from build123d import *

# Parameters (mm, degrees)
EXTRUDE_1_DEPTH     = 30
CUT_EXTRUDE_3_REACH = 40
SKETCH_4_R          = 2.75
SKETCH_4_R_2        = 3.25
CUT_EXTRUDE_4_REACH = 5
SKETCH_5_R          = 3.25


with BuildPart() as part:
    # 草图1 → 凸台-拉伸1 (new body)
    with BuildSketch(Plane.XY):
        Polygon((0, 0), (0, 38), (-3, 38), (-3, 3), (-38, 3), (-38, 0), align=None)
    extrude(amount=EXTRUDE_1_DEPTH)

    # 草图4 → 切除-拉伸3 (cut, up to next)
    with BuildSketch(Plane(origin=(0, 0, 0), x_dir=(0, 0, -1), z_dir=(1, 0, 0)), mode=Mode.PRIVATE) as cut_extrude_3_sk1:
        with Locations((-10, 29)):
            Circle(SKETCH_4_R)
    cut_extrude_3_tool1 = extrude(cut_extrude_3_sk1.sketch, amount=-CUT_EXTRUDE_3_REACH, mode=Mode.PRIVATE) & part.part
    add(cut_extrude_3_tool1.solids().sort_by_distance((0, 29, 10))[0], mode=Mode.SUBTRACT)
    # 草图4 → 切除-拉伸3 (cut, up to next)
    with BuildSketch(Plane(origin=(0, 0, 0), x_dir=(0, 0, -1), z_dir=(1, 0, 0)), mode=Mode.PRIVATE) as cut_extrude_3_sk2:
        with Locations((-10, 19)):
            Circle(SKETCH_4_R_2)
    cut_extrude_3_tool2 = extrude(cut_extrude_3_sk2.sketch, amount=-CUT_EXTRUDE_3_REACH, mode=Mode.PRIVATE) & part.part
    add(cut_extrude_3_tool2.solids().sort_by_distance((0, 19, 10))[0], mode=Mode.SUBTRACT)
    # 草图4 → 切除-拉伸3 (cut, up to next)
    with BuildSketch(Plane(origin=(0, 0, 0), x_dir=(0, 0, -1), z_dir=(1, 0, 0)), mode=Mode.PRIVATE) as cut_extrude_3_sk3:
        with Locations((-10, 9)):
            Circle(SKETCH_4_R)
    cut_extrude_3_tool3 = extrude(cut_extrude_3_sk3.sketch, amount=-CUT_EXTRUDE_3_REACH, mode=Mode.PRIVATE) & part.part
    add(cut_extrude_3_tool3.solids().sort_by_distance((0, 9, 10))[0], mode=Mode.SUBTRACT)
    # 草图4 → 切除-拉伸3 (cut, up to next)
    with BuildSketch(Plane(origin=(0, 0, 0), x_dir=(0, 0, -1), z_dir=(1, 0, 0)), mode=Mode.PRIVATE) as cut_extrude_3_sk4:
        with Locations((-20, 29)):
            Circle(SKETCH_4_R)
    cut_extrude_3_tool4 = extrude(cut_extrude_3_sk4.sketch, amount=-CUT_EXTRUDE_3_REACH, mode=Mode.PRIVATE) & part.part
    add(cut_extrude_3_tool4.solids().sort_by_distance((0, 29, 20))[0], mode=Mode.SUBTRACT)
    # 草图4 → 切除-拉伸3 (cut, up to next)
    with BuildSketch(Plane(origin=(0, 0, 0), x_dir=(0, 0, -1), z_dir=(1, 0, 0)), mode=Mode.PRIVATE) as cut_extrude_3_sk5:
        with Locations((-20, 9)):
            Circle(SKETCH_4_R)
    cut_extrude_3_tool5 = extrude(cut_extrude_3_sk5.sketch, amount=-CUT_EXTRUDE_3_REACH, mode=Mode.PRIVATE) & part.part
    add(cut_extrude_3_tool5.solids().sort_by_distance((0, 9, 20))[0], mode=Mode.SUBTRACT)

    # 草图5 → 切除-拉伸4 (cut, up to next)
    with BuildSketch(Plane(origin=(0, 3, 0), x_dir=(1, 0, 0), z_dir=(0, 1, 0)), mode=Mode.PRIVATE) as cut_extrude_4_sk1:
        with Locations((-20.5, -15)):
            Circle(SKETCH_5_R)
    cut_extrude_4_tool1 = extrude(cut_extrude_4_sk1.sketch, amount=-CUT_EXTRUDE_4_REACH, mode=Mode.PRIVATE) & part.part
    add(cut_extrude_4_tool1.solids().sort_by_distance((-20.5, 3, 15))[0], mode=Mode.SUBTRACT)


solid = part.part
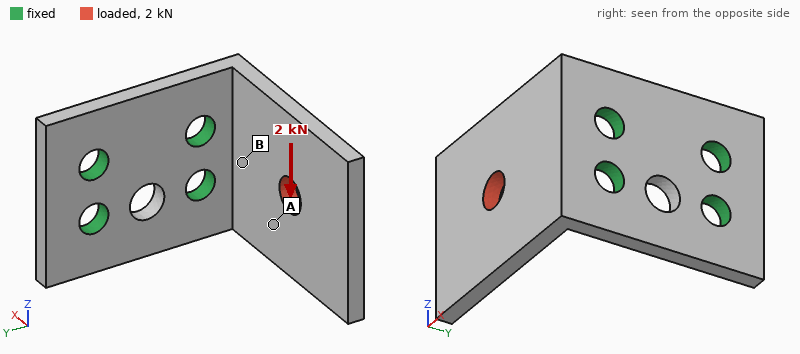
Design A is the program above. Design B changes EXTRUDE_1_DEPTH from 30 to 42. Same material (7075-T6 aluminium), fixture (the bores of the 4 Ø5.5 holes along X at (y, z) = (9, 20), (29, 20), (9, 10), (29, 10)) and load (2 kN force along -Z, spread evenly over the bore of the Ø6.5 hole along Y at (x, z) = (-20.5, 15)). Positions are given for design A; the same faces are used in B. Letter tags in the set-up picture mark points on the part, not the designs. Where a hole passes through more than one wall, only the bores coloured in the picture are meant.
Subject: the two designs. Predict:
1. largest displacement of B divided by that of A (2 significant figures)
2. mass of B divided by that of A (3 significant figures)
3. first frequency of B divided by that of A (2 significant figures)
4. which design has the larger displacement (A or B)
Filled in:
1.1
1.43
0.96
B
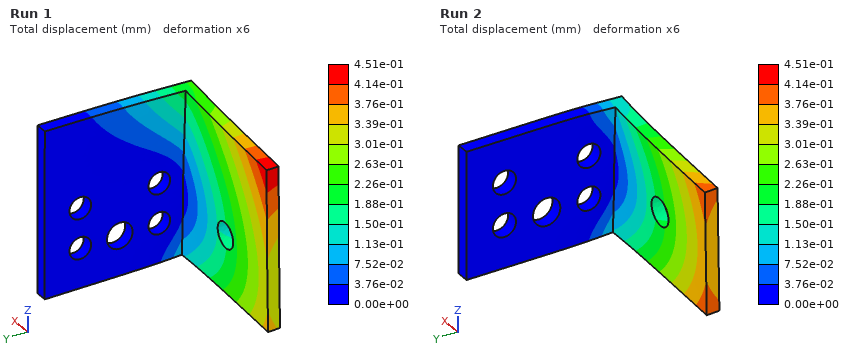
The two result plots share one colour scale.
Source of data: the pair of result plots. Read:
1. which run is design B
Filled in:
Run 1
